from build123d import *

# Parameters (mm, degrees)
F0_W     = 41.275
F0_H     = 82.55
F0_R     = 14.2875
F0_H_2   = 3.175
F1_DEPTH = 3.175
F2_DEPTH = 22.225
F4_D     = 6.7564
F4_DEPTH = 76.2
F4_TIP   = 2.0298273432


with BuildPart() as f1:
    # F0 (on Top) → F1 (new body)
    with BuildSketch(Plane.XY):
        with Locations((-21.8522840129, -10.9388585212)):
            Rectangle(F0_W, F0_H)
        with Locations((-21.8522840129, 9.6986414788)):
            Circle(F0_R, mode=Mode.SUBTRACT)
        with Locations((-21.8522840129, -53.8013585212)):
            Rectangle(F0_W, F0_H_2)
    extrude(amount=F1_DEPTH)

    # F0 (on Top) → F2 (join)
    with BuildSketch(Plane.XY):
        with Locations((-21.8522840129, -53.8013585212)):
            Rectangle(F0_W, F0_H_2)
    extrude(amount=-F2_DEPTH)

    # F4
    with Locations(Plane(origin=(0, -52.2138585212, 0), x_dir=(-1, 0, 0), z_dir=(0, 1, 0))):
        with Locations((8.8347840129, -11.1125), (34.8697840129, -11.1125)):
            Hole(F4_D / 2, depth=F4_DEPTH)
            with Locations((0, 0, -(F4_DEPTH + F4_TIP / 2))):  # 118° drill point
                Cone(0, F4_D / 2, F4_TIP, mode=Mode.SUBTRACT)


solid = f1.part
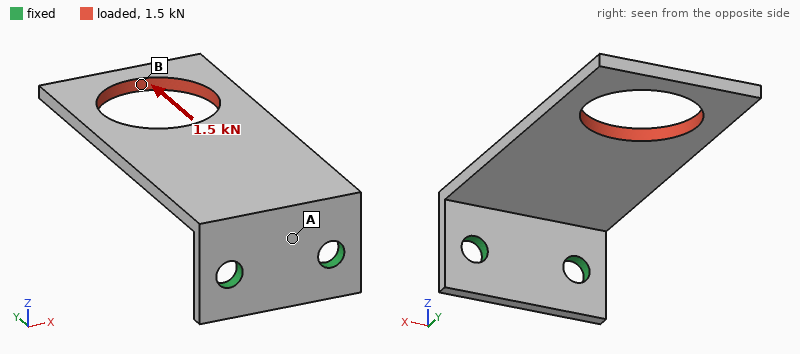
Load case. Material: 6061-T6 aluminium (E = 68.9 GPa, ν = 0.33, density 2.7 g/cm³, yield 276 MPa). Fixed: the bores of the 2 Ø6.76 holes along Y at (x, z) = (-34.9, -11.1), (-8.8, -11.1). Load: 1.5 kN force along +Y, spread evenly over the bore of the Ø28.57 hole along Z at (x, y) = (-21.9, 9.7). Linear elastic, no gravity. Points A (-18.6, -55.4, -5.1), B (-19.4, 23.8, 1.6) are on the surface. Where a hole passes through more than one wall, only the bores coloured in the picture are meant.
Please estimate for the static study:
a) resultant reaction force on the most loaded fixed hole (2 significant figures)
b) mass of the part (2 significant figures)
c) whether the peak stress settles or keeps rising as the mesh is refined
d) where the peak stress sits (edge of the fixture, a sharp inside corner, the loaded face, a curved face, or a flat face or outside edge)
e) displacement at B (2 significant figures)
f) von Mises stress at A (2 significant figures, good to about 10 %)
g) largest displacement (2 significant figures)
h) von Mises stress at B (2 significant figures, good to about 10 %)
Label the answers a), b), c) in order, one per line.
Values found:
a) 750 N
b) 32 g
c) keeps rising
d) edge of the fixture
e) 0.87 mm
f) 84 MPa
g) 0.95 mm
h) 31 MPa
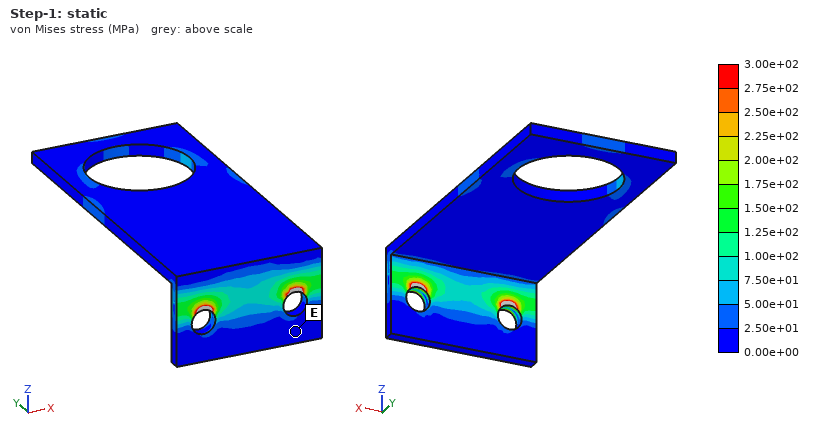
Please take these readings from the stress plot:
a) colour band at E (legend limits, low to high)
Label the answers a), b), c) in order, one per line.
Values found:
a) 0.00e+00 to 2.50e+01 MPa
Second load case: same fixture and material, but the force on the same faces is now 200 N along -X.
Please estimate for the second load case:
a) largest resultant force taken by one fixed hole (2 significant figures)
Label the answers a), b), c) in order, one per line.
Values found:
a) 460 N
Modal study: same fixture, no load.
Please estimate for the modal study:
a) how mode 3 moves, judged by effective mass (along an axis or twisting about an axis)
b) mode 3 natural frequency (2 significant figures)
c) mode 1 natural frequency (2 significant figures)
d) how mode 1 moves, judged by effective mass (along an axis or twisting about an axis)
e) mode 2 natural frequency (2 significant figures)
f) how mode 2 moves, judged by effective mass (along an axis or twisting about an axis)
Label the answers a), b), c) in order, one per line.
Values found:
a) along X
b) 1700 Hz
c) 370 Hz
d) along Z
e) 1400 Hz
f) along X
